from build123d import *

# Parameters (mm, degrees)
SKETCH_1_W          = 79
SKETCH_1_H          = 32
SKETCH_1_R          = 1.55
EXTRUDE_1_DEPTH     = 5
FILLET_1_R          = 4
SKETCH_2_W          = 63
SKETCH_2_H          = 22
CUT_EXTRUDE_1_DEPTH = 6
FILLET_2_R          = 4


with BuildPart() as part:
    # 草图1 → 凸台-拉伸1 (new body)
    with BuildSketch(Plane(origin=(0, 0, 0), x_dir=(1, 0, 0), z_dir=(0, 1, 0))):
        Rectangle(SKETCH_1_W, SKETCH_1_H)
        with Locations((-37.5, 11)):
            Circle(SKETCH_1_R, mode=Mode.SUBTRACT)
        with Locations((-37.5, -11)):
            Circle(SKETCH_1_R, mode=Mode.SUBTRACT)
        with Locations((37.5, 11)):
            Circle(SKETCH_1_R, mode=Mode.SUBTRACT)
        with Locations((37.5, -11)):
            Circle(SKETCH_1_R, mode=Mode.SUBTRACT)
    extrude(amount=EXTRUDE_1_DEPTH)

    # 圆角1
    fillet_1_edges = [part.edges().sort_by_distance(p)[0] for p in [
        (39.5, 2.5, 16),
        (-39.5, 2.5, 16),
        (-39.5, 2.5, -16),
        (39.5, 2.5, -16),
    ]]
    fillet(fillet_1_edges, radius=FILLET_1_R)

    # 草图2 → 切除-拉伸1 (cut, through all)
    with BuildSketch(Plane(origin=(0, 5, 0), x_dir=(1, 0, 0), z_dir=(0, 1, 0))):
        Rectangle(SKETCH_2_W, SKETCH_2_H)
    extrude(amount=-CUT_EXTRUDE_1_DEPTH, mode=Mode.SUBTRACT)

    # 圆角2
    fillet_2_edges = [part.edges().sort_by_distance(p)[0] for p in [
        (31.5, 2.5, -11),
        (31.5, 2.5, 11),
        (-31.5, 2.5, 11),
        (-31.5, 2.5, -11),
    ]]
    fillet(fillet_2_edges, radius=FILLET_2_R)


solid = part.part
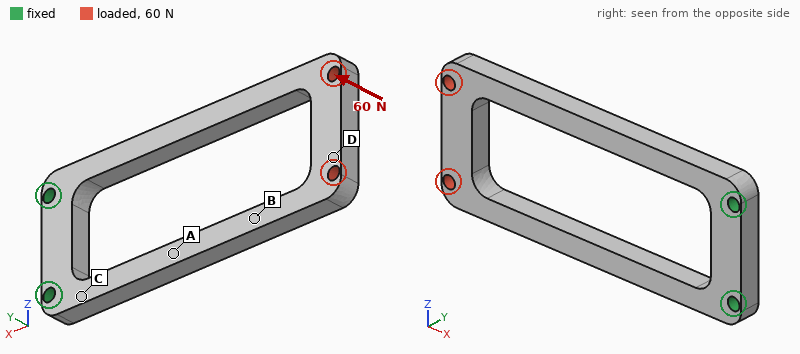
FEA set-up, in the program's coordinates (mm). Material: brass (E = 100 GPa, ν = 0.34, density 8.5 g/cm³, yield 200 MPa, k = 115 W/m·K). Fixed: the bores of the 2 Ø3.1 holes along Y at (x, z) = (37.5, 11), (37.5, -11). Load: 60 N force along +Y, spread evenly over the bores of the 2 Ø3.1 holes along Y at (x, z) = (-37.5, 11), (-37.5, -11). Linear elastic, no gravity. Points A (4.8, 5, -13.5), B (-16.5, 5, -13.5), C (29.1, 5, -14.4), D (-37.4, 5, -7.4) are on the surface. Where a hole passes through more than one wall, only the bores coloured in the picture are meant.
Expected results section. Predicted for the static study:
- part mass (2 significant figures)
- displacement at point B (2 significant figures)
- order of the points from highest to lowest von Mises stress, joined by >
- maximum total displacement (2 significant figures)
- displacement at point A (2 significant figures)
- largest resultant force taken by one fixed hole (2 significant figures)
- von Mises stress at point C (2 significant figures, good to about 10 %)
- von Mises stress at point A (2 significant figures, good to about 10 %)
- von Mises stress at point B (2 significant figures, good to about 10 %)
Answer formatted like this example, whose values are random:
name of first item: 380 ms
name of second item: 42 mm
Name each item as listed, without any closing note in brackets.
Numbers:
part mass: 47 g
displacement at point B: 0.43 mm
order of the points from highest to lowest von Mises stress, joined by >: C > A > B > D
maximum total displacement: 0.77 mm
displacement at point A: 0.17 mm
largest resultant force taken by one fixed hole: 30 N
von Mises stress at point C: 86 MPa
von Mises stress at point A: 61 MPa
von Mises stress at point B: 30 MPa
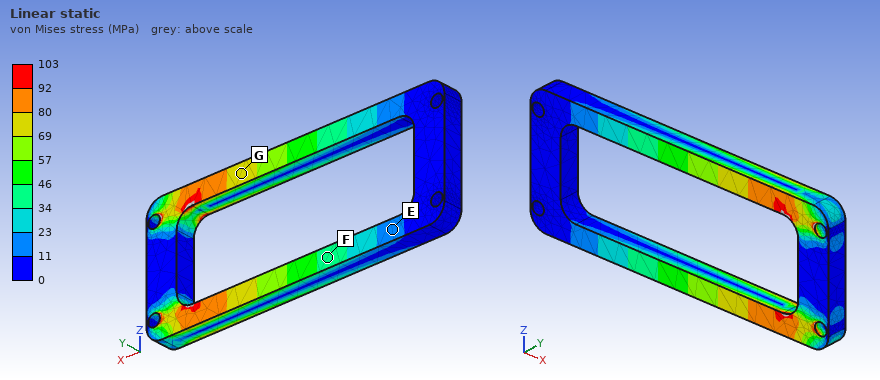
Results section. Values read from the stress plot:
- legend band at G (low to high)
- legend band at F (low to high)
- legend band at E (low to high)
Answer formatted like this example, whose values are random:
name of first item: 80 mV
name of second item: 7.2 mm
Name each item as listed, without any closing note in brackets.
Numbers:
legend band at G: 69 to 80 MPa
legend band at F: 34 to 46 MPa
legend band at E: 11 to 23 MPa
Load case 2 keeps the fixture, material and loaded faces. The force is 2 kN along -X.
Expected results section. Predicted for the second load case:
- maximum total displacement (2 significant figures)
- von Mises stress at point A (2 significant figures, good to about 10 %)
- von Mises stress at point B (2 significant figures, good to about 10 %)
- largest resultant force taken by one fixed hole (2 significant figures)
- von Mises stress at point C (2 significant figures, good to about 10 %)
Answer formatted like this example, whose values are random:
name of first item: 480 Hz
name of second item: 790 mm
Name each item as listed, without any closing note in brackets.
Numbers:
maximum total displacement: 40 µm
von Mises stress at point A: 40 MPa
von Mises stress at point B: 40 MPa
largest resultant force taken by one fixed hole: 1.0 kN
von Mises stress at point C: 41 MPa
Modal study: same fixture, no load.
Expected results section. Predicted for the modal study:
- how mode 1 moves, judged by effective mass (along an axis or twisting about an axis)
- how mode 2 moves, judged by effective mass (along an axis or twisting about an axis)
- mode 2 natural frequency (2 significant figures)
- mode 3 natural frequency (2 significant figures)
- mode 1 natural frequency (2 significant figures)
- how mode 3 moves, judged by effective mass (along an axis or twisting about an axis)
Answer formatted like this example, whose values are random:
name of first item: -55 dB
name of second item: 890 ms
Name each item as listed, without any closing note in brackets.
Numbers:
how mode 1 moves, judged by effective mass: along Y
how mode 2 moves, judged by effective mass: along Z
mode 2 natural frequency: 720 Hz
mode 3 natural frequency: 1200 Hz
mode 1 natural frequency: 380 Hz
how mode 3 moves, judged by effective mass: twisting about X
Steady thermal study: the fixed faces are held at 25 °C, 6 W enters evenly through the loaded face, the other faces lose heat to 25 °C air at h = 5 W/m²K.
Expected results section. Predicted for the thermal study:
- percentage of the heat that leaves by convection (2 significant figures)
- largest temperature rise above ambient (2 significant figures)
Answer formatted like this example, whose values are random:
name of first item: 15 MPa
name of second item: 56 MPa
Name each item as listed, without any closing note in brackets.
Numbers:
percentage of the heat that leaves by convection: 11 %
largest temperature rise above ambient: 68 K
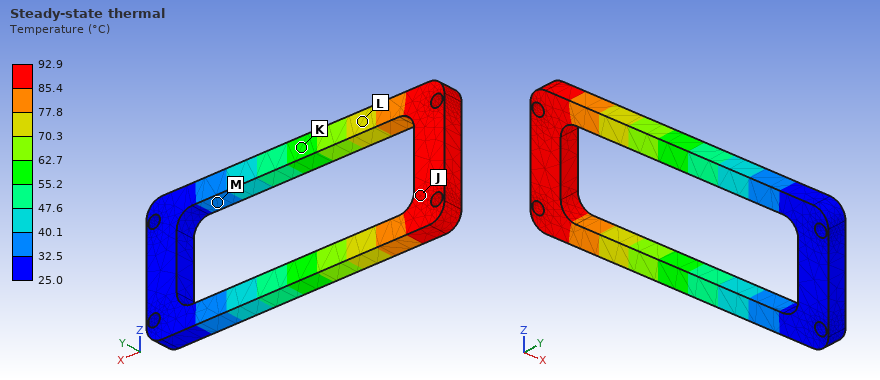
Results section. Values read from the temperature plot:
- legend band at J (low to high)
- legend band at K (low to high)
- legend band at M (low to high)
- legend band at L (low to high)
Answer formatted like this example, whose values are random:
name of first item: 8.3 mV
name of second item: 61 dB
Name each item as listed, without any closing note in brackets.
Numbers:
legend band at J: 85.4 to 92.9 °C
legend band at K: 55.2 to 62.7 °C
legend band at M: 32.5 to 40.1 °C
legend band at L: 70.3 to 77.8 °C
